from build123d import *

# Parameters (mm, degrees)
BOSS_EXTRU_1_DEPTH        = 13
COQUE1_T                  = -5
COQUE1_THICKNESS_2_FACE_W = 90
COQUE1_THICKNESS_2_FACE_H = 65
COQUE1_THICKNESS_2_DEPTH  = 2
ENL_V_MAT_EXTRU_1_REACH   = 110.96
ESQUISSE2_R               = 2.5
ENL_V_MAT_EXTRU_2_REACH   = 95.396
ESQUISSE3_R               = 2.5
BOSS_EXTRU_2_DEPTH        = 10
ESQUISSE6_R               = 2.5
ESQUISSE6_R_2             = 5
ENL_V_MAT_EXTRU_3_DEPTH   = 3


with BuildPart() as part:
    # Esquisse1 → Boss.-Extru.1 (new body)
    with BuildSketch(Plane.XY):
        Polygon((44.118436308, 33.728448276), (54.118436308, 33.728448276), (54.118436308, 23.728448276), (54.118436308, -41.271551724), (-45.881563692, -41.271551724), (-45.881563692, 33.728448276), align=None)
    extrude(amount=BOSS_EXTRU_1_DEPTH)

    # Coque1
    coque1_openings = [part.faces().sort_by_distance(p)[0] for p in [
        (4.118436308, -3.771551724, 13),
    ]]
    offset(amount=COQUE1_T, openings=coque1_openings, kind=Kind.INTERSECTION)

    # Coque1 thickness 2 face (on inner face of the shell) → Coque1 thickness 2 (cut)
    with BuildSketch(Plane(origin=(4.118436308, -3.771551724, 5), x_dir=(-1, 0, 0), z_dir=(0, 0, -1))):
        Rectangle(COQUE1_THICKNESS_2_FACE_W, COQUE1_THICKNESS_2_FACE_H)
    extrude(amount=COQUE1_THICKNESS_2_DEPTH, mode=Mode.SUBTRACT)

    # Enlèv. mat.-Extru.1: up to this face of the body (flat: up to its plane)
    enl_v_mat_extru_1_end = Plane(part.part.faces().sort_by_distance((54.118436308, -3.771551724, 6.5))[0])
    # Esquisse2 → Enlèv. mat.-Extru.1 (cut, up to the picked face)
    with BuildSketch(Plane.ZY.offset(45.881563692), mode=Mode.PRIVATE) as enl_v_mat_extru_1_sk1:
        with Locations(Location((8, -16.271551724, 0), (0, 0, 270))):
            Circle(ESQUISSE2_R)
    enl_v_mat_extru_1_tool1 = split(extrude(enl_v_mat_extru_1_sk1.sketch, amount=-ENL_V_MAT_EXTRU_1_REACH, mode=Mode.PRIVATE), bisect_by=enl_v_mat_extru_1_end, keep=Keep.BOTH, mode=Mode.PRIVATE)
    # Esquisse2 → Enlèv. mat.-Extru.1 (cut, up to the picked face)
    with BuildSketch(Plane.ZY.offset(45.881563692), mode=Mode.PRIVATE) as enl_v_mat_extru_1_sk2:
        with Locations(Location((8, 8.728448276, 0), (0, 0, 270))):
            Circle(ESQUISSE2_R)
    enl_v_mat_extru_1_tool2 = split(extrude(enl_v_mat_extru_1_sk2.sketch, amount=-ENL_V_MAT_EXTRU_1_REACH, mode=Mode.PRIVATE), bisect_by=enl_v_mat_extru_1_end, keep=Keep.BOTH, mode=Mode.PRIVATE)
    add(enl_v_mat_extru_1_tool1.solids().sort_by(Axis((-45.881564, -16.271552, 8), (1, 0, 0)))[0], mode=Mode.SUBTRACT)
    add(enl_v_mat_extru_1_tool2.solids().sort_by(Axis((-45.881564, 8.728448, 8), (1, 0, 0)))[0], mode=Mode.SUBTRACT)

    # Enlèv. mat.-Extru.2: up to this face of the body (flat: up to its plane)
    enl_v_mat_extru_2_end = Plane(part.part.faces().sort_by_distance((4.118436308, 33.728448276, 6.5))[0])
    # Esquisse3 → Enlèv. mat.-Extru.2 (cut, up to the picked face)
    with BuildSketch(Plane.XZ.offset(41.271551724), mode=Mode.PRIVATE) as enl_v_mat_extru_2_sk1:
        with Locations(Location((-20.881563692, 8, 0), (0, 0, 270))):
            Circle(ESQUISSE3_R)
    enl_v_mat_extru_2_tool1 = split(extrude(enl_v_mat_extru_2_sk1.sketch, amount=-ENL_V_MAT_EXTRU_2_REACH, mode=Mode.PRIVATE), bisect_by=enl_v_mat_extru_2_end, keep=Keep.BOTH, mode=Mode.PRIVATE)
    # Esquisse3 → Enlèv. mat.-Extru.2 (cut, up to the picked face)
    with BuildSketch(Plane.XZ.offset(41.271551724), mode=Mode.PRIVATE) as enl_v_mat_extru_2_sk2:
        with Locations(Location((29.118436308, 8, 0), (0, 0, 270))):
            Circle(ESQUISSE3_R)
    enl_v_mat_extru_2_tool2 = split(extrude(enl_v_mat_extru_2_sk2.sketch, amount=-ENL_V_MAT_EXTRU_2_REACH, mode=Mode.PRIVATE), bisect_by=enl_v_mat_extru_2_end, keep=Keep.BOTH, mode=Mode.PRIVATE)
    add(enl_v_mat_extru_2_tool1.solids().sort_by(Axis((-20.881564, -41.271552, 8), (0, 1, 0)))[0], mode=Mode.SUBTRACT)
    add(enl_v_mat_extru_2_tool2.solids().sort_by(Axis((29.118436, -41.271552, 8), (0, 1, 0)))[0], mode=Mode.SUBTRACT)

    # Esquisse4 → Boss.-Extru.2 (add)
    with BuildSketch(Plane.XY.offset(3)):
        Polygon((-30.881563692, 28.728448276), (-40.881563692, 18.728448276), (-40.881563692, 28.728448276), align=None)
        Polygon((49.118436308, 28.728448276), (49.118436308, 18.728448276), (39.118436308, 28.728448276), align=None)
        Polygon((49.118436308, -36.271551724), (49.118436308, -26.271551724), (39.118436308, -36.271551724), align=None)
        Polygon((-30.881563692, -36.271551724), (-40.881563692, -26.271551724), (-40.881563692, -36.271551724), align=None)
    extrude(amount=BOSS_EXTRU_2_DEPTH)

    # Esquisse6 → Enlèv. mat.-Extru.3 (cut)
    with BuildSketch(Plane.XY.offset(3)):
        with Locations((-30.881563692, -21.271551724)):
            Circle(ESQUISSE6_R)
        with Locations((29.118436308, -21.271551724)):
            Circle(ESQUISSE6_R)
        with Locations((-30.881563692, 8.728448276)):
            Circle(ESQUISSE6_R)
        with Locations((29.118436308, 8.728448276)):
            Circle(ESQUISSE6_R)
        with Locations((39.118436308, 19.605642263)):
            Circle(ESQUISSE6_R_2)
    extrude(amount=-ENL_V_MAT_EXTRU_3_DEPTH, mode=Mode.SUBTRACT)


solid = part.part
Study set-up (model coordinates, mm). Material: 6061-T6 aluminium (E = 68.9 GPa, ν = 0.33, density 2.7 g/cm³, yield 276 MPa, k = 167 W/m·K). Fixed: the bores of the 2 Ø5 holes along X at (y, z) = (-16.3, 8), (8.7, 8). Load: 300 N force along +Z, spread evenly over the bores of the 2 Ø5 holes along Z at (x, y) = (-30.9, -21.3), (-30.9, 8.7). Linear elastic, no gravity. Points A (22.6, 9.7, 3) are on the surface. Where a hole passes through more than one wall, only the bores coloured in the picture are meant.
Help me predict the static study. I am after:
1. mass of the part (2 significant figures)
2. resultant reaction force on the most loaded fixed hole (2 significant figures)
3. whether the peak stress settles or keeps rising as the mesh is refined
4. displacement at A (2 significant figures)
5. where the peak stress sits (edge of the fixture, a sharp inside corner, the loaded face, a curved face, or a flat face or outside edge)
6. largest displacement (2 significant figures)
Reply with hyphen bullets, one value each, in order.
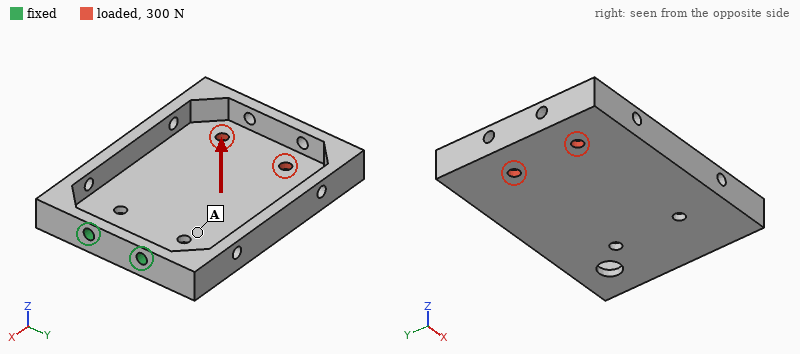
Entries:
- 110 g
- 370 N
- keeps rising
- 0.22 mm
- edge of the fixture
- 0.99 mm
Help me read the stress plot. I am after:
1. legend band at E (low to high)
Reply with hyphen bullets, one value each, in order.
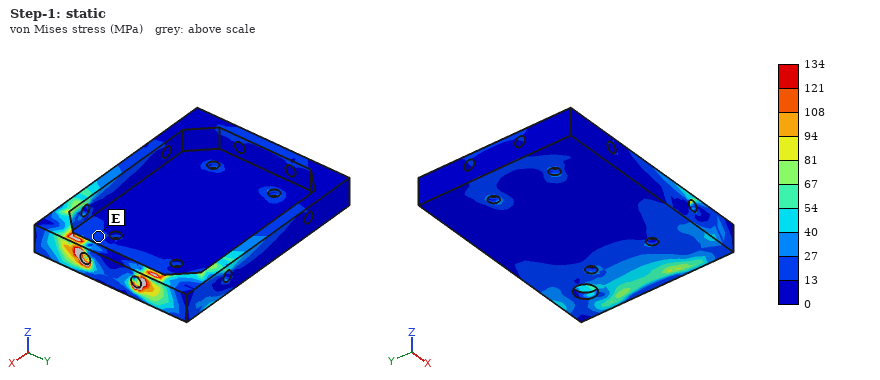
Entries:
- 13 to 27 MPa
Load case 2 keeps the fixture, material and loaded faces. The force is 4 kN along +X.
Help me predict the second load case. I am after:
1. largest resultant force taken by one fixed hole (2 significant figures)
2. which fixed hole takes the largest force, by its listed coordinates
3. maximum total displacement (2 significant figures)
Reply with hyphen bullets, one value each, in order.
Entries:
- 2.3 kN
- (-16.3, 8)
- 0.33 mm
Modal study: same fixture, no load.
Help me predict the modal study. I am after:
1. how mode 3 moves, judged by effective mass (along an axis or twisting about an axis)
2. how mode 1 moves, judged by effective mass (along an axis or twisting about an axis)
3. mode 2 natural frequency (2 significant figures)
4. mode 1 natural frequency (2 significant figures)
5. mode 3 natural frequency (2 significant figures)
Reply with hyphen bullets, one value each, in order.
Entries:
- along Y
- along Z
- 860 Hz
- 430 Hz
- 1600 Hz
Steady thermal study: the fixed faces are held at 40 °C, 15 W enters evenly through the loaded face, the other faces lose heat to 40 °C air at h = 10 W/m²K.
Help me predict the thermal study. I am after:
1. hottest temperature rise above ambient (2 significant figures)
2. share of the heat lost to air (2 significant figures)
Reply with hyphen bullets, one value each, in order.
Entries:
- 27 K
- 21 %
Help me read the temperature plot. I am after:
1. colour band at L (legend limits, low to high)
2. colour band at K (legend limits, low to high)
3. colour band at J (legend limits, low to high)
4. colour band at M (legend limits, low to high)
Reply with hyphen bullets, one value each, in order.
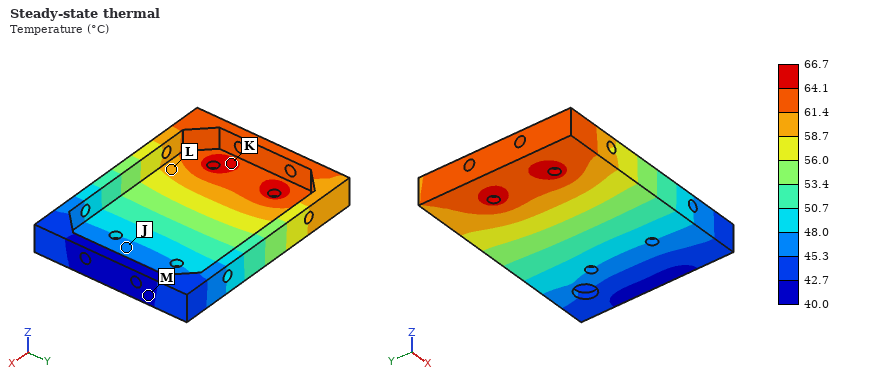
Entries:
- 58.7 to 61.4 °C
- 64.1 to 66.7 °C
- 45.3 to 48.0 °C
- 40.0 to 42.7 °C
